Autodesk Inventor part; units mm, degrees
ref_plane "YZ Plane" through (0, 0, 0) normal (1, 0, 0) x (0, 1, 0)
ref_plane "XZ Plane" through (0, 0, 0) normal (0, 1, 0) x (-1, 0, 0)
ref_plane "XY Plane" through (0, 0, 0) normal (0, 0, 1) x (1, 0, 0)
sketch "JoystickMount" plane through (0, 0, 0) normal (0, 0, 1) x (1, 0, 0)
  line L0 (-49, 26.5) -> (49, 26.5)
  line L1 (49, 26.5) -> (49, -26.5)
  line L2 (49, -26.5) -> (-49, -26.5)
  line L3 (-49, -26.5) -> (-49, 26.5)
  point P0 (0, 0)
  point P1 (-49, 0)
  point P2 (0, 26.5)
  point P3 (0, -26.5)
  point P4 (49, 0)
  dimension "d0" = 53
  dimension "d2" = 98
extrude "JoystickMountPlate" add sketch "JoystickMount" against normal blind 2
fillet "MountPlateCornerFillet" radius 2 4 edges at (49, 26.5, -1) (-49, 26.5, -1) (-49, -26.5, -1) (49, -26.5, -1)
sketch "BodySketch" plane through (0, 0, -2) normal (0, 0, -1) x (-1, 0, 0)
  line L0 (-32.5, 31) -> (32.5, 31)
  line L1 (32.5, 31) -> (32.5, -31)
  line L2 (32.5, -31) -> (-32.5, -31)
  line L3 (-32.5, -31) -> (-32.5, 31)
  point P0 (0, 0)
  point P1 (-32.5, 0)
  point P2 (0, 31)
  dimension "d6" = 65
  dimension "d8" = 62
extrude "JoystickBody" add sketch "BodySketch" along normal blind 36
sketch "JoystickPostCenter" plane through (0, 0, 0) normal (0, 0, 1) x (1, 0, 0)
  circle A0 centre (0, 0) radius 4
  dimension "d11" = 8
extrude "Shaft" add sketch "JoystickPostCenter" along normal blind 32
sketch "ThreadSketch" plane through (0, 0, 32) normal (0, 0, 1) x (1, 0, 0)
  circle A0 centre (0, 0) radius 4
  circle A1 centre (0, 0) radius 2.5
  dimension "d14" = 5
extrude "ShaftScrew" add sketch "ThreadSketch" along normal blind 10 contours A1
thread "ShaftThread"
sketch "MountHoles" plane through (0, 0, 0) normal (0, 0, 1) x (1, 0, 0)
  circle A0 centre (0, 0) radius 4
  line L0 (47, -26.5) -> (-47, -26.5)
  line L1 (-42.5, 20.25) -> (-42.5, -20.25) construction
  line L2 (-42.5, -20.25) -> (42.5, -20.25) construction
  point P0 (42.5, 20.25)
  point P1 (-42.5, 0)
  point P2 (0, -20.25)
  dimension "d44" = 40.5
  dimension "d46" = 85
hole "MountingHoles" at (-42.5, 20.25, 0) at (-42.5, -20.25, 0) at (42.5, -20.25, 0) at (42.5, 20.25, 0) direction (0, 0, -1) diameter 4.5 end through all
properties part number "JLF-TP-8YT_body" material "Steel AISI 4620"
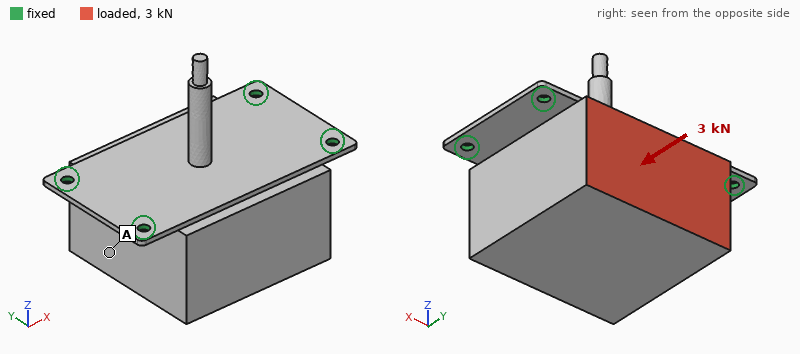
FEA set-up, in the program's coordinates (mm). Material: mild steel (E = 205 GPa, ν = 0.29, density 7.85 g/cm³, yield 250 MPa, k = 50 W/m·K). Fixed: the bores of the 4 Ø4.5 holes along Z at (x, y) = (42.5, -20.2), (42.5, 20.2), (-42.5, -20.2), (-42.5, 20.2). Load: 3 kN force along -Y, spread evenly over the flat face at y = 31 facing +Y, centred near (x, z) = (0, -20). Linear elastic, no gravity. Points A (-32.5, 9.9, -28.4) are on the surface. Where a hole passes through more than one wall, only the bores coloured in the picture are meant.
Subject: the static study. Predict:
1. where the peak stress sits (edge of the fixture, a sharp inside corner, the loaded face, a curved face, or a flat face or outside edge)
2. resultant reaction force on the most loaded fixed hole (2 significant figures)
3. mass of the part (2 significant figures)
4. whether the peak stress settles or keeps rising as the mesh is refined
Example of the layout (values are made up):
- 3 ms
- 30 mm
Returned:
- edge of the fixture
- 1.2 kN
- 1.2 kg
- keeps rising
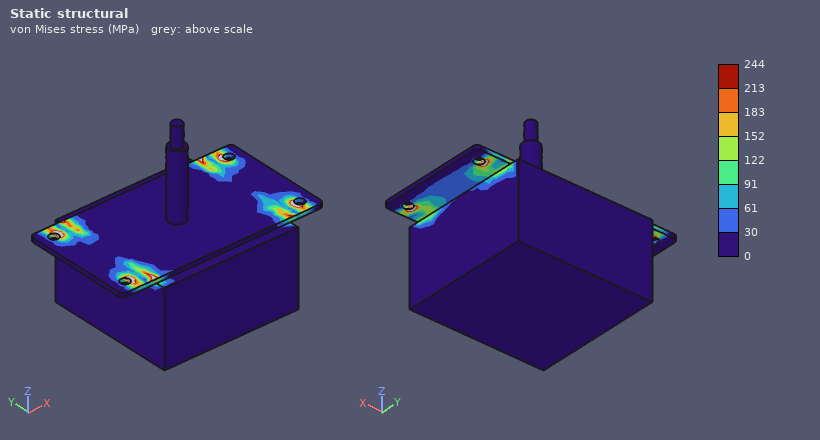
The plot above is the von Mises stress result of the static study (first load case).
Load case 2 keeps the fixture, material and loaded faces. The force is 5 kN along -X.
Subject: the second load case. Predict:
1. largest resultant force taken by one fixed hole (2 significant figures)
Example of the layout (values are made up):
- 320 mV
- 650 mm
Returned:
- 1.9 kN
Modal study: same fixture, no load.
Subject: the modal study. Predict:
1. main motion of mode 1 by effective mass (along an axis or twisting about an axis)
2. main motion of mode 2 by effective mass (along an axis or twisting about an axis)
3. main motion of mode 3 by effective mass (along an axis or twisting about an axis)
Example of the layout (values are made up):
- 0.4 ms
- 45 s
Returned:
- along Y
- along Z
- along X
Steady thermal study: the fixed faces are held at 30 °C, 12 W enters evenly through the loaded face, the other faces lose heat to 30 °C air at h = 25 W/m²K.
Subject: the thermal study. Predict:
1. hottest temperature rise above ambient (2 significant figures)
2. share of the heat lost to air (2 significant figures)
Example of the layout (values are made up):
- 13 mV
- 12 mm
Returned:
- 14 K
- 43 %
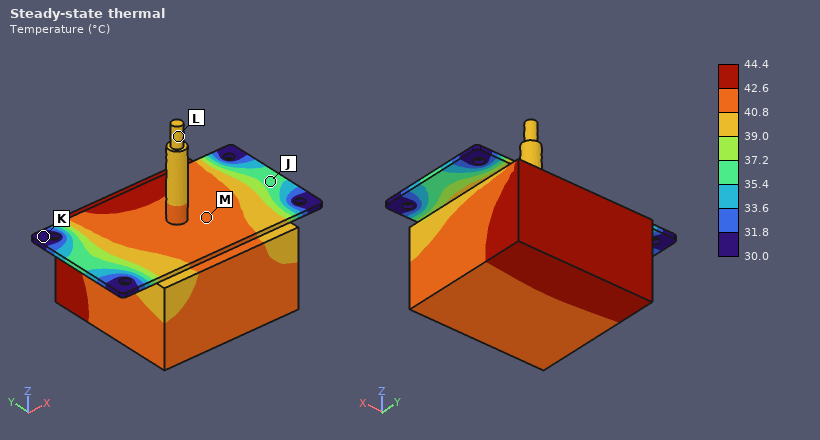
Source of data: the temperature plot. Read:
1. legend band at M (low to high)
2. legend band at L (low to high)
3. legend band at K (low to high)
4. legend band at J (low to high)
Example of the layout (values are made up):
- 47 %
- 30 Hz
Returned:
- 40.8 to 42.6 °C
- 39.0 to 40.8 °C
- 30.0 to 31.8 °C
- 35.4 to 37.2 °C
